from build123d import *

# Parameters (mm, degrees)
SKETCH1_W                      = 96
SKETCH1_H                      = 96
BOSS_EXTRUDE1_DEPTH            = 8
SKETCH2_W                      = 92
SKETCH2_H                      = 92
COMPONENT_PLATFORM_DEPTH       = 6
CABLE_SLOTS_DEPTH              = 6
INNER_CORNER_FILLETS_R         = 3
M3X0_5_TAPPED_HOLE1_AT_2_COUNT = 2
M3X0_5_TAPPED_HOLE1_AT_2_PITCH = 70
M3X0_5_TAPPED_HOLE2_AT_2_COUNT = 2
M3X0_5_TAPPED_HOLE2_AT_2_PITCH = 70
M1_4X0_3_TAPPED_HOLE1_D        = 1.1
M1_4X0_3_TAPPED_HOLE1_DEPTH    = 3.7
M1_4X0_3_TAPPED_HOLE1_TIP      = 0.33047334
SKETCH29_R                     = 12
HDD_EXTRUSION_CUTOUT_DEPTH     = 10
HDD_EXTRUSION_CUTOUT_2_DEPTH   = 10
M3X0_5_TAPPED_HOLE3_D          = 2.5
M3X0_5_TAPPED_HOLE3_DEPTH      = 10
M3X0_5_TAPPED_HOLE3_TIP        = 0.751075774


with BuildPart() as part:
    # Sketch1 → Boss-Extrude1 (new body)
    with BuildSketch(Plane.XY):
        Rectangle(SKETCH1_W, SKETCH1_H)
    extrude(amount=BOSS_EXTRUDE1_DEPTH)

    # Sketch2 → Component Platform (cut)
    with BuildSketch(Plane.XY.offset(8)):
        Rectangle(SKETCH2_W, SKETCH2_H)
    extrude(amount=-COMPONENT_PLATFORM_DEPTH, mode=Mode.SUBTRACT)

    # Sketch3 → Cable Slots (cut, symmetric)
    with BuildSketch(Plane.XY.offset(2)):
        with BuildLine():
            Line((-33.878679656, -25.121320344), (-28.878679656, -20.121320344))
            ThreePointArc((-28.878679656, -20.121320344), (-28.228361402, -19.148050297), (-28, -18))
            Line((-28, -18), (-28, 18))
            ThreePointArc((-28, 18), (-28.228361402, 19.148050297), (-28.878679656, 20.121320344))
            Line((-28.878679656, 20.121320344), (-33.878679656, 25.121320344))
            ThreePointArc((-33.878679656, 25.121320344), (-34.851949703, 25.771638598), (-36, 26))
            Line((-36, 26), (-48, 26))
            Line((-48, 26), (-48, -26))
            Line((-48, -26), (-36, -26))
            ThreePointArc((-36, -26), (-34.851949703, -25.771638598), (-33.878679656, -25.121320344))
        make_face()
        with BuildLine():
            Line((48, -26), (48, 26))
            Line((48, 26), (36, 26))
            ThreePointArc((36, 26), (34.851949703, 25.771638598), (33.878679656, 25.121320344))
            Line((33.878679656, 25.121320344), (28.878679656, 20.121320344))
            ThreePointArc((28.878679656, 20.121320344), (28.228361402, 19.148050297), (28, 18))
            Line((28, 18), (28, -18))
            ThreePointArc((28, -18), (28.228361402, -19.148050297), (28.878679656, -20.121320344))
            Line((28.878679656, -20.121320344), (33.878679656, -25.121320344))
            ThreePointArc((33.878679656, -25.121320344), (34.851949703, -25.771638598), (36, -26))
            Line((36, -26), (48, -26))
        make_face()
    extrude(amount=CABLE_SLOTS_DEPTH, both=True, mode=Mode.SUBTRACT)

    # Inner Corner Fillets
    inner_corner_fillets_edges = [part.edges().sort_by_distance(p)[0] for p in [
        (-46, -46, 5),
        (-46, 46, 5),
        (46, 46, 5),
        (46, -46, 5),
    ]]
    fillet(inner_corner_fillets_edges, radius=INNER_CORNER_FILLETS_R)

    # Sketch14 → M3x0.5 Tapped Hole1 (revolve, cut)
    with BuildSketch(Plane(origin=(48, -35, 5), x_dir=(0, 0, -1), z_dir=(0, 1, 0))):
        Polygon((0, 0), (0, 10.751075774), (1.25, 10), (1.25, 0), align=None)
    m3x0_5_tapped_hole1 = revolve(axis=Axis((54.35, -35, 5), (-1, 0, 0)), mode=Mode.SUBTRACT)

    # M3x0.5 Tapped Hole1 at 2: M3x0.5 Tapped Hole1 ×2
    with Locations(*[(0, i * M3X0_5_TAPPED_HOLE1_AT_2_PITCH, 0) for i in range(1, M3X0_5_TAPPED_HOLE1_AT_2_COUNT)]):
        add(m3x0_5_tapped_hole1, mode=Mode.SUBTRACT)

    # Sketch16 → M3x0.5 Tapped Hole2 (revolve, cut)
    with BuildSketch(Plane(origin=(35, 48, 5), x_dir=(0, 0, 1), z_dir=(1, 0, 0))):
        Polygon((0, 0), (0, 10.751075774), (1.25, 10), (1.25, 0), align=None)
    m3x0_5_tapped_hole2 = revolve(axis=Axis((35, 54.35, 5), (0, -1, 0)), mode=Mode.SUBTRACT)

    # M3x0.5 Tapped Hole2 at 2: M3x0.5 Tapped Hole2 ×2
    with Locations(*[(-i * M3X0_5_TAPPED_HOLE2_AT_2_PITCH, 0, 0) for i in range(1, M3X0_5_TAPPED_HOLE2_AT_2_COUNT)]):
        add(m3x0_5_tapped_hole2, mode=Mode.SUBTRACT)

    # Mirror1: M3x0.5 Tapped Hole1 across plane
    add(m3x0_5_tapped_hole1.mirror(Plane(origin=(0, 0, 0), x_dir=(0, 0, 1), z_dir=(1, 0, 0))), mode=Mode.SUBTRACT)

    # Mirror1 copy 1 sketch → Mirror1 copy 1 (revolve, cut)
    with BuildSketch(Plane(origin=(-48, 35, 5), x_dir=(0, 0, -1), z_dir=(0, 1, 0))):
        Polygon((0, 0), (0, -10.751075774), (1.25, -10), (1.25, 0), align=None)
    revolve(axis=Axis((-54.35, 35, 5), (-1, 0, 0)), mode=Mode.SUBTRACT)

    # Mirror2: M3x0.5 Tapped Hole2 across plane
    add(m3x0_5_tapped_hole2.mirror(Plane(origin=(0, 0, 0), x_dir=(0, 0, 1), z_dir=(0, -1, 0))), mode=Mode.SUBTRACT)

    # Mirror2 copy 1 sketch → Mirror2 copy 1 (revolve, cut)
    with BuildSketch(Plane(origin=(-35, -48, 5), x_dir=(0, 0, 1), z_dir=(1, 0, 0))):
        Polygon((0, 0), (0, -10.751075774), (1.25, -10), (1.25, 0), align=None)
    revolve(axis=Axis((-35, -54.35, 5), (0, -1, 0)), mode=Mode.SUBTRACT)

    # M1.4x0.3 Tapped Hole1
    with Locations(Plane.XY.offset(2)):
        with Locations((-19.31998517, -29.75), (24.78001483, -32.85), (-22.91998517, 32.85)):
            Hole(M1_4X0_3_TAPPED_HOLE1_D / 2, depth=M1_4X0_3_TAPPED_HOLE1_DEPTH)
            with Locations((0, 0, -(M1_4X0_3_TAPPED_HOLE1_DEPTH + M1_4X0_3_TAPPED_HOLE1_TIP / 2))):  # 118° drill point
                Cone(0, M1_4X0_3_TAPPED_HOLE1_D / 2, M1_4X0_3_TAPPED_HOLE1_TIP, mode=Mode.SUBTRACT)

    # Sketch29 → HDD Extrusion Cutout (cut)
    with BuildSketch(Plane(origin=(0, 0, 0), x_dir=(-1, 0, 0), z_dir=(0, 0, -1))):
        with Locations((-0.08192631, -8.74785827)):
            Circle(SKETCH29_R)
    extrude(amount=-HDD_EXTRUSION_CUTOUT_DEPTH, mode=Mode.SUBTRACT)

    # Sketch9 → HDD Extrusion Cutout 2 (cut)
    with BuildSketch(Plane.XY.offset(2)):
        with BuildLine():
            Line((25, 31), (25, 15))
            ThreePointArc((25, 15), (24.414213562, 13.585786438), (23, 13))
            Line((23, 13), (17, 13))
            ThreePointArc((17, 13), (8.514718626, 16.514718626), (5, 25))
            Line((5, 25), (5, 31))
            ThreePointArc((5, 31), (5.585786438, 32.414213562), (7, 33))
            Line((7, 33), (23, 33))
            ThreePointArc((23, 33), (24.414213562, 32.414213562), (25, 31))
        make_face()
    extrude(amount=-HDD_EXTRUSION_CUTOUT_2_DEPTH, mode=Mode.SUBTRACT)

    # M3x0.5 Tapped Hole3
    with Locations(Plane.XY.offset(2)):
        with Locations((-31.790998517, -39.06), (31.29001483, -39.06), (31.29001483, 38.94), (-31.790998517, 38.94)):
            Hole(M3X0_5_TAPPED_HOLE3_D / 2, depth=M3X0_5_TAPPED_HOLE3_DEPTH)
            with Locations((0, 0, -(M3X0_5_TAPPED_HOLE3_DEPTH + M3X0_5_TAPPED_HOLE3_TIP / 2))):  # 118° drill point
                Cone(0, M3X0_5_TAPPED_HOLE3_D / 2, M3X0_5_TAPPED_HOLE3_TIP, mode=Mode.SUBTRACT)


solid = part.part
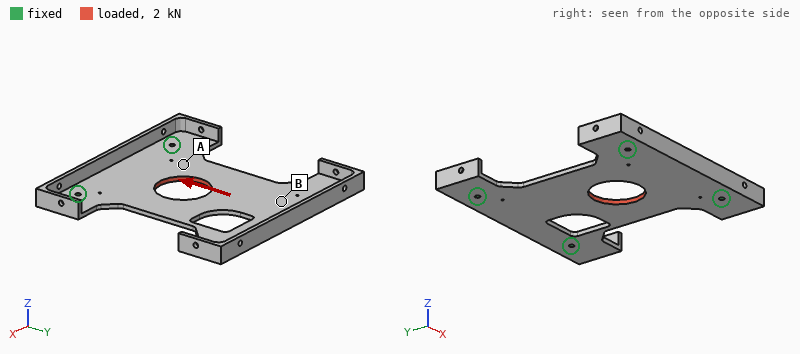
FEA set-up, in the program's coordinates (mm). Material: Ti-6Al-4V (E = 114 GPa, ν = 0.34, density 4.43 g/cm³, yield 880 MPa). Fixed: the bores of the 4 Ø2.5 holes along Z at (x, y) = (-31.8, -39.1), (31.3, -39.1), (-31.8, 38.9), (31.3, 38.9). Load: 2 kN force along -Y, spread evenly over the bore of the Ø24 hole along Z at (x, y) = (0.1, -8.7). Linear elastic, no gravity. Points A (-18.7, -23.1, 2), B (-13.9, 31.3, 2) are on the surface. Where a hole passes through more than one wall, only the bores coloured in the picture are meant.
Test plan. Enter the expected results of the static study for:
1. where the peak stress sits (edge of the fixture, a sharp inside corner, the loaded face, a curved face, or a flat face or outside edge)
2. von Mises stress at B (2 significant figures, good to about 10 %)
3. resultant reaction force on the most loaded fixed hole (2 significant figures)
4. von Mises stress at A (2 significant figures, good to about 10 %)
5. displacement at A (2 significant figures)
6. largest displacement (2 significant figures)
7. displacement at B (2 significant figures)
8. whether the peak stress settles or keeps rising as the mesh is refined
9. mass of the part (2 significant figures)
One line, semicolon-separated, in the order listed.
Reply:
edge of the fixture; 5.4 MPa; 720 N; 14 MPa; 6.1 µm; 13 µm; 6.0 µm; keeps rising; 71 g
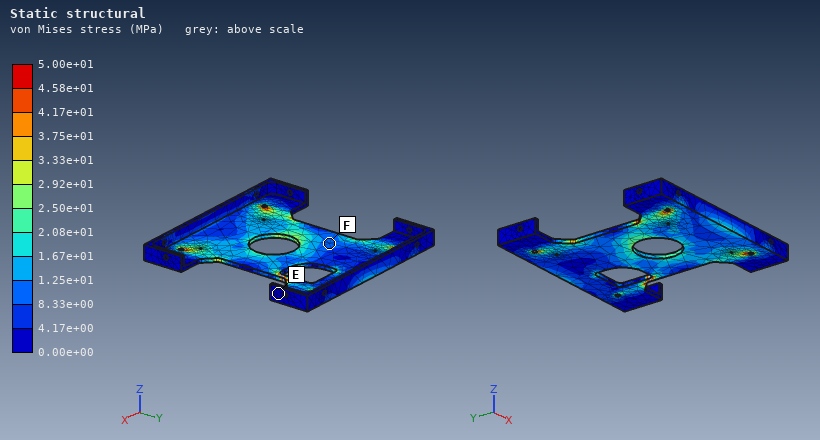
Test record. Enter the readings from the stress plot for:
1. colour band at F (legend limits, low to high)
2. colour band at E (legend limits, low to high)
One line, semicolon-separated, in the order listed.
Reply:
8.33e+00 to 1.25e+01 MPa; 0.00e+00 to 4.17e+00 MPa
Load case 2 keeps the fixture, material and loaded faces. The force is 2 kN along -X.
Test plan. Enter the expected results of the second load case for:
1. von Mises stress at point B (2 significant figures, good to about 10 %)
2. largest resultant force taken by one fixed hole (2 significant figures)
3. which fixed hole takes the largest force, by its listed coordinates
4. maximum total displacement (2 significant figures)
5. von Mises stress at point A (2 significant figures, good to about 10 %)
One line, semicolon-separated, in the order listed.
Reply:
11 MPa; 860 N; (-31.8, -39.1); 14 µm; 18 MPa
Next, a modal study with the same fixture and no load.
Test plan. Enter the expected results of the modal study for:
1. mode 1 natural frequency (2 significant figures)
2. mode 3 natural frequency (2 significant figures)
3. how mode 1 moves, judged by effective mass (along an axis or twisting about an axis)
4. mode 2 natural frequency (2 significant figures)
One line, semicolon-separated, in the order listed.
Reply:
1400 Hz; 3100 Hz; along Z; 2400 Hz
